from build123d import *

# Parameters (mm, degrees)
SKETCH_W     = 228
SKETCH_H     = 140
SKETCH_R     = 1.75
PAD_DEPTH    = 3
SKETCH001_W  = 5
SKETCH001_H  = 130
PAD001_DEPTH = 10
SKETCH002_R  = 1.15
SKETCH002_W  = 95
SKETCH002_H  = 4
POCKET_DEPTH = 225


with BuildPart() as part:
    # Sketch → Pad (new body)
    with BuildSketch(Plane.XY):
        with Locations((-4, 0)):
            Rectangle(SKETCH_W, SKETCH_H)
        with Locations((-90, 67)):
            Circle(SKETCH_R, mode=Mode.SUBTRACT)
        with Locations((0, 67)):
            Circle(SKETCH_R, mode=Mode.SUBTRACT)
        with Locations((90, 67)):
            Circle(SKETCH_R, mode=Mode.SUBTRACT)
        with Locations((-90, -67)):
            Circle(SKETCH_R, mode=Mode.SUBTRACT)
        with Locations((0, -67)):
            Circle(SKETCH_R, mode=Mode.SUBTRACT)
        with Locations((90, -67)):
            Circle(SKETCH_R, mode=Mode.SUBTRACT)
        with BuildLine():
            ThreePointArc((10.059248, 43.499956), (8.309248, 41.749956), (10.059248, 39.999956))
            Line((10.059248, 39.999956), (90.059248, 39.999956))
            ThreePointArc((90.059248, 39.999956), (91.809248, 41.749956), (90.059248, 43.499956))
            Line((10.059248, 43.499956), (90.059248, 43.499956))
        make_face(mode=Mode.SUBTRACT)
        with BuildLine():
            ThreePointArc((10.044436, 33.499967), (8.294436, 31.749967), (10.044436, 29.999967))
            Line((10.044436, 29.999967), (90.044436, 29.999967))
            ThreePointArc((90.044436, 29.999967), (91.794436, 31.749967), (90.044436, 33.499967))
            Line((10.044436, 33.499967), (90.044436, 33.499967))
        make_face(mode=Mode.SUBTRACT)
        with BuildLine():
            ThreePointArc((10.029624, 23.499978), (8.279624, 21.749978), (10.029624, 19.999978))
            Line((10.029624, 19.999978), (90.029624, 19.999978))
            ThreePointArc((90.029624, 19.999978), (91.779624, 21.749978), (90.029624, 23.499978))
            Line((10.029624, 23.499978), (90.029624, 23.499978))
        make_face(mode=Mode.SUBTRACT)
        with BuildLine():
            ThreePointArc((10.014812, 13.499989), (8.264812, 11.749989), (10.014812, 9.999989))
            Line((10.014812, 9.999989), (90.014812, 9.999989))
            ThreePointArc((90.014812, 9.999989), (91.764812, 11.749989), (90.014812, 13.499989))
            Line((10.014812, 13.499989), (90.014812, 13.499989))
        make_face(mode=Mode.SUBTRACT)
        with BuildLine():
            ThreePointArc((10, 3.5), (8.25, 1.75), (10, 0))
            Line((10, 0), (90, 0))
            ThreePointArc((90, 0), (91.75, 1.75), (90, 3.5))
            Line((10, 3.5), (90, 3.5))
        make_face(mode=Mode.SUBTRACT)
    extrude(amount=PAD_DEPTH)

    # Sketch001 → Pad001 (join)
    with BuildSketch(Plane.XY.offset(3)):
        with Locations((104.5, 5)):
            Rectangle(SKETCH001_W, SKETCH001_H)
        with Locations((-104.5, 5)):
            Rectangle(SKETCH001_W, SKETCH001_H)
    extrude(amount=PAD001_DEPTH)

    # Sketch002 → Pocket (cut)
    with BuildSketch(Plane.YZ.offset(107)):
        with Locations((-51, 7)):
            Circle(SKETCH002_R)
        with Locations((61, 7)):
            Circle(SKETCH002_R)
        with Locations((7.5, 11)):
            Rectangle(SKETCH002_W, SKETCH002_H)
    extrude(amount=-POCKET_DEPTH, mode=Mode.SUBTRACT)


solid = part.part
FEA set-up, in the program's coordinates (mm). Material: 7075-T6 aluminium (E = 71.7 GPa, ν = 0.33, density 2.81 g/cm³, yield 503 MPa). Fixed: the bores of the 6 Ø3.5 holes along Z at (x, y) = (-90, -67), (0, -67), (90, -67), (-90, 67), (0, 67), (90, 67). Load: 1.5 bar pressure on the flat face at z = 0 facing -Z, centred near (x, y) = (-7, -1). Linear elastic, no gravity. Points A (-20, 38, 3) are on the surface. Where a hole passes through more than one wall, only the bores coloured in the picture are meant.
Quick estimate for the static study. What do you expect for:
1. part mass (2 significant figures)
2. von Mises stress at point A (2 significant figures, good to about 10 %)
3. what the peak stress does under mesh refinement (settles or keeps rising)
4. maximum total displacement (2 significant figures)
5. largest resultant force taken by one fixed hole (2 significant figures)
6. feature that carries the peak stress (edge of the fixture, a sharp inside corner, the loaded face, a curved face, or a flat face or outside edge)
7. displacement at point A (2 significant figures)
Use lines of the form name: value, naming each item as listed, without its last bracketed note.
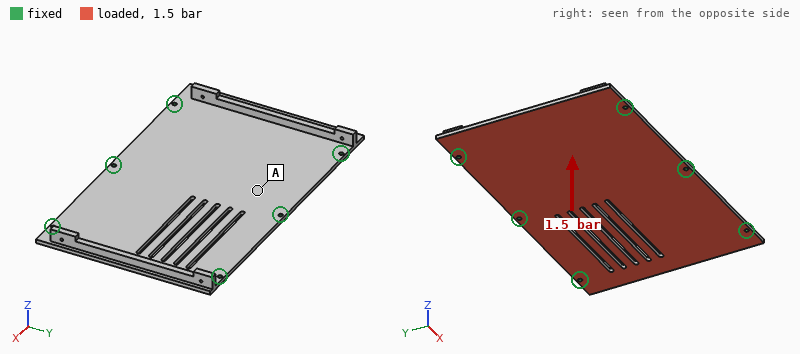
part mass: 280 g
von Mises stress at point A: 58 MPa
what the peak stress does under mesh refinement: keeps rising
maximum total displacement: 1.7 mm
largest resultant force taken by one fixed hole: 1.1 kN
feature that carries the peak stress: edge of the fixture
displacement at point A: 0.80 mm
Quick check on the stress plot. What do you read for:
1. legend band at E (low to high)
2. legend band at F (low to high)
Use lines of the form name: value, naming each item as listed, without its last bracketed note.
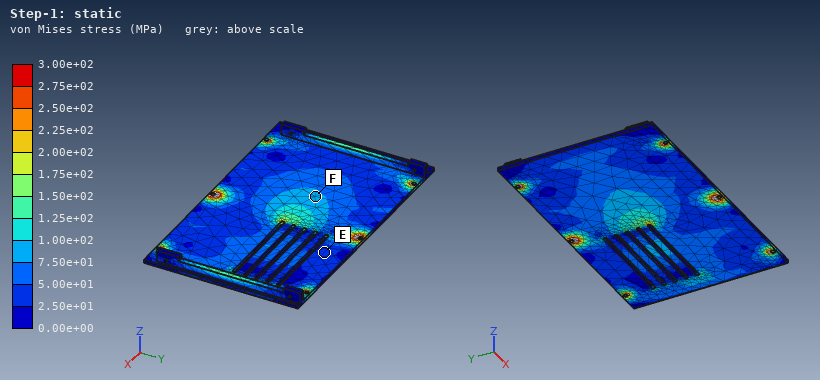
legend band at E: 2.50e+01 to 5.00e+01 MPa
legend band at F: 7.50e+01 to 1.00e+02 MPa
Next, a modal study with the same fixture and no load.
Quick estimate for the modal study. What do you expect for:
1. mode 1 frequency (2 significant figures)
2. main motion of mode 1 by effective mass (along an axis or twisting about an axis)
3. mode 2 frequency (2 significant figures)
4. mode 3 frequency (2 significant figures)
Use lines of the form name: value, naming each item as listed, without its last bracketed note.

mode 1 frequency: 660 Hz
main motion of mode 1 by effective mass: along Z
mode 2 frequency: 920 Hz
mode 3 frequency: 1100 Hz
